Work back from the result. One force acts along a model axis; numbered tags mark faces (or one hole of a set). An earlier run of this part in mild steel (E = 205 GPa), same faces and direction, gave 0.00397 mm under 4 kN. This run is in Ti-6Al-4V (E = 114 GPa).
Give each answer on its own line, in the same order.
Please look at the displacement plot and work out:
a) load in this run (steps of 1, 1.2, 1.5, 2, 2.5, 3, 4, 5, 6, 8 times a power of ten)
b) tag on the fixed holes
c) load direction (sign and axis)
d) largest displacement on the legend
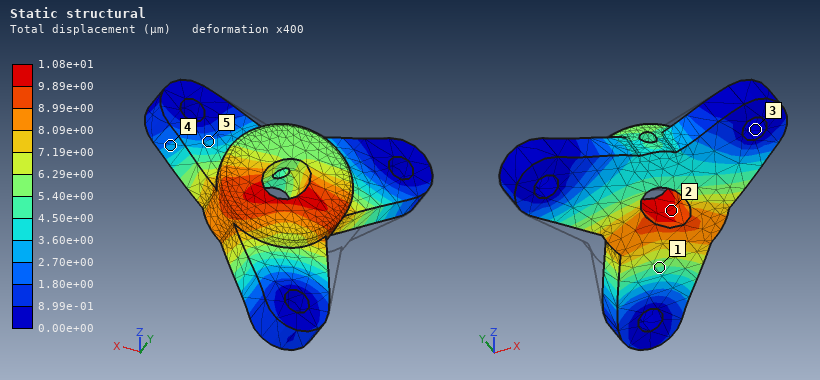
6 kN
3
+X
1.08e+01 µm
